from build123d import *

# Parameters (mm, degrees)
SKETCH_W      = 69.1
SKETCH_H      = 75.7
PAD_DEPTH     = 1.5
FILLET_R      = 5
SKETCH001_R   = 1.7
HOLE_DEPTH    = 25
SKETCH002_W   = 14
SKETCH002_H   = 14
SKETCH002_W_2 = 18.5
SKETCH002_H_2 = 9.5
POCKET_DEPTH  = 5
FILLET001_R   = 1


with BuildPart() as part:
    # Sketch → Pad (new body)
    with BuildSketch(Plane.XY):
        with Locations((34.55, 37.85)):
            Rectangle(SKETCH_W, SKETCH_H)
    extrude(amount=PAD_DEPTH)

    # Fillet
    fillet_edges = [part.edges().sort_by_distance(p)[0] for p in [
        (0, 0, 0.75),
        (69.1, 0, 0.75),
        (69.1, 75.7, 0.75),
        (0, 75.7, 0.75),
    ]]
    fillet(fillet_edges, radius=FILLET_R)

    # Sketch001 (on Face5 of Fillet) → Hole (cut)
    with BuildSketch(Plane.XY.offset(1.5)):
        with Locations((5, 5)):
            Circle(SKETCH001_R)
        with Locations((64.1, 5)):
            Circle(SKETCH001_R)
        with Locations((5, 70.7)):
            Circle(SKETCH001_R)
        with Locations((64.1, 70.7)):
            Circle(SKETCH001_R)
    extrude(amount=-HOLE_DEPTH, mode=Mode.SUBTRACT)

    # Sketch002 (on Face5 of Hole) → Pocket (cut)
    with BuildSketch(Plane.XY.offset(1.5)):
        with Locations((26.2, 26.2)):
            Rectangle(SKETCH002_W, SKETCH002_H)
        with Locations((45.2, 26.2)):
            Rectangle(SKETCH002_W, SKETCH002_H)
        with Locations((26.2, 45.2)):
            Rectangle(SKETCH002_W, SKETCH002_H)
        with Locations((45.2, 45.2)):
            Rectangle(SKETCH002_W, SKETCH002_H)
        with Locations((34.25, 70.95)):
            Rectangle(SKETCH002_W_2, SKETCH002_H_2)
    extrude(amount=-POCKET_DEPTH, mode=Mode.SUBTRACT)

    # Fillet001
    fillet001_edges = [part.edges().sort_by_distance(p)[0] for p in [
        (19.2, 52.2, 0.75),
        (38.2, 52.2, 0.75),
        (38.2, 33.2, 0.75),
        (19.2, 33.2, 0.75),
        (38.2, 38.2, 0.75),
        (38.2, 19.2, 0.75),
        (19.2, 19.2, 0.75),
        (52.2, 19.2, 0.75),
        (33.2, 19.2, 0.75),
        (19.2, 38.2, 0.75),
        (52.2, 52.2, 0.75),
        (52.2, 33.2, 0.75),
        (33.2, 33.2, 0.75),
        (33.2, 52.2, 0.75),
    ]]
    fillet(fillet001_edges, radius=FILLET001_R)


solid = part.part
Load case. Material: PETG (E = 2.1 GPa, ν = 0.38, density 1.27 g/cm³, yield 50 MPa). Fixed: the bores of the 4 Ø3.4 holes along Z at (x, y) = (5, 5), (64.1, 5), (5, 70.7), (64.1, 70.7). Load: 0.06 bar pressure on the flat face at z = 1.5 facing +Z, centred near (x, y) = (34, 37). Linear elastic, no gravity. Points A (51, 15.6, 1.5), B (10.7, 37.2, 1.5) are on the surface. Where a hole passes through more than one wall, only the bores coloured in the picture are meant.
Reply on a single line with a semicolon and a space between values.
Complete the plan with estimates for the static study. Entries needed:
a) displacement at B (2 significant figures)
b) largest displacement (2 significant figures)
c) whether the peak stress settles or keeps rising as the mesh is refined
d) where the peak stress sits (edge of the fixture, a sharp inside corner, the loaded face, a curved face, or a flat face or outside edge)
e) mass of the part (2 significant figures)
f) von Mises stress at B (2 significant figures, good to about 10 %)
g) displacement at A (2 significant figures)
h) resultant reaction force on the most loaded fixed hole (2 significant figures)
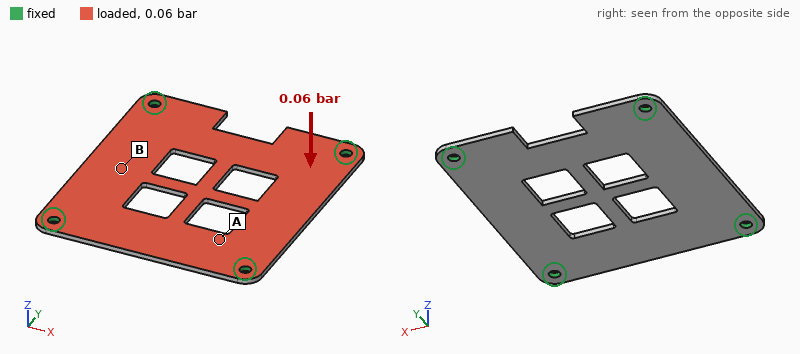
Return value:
0.69 mm; 1.1 mm; keeps rising; edge of the fixture; 8.0 g; 3.3 MPa; 0.44 mm; 6.6 N
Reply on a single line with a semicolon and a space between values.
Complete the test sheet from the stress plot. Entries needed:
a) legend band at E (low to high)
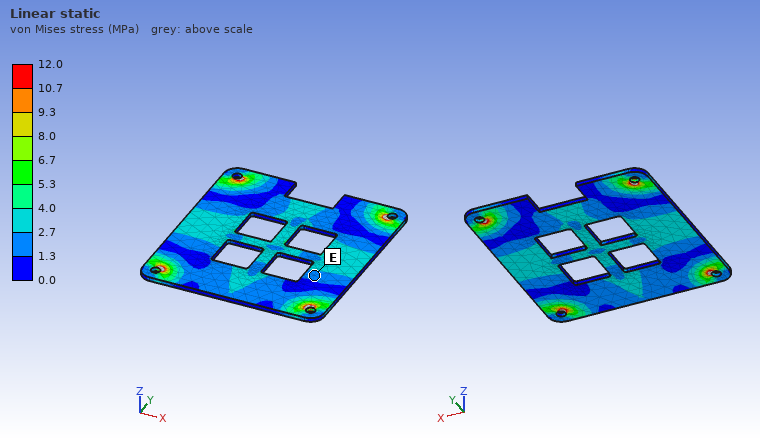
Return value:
1.3 to 2.7 MPa
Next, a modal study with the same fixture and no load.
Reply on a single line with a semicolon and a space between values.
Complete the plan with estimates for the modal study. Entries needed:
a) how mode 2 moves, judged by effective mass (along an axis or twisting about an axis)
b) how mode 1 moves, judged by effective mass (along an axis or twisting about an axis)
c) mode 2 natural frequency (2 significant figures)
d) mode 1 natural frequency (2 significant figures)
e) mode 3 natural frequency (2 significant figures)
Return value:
twisting about Y; along Z; 530 Hz; 360 Hz; 610 Hz
